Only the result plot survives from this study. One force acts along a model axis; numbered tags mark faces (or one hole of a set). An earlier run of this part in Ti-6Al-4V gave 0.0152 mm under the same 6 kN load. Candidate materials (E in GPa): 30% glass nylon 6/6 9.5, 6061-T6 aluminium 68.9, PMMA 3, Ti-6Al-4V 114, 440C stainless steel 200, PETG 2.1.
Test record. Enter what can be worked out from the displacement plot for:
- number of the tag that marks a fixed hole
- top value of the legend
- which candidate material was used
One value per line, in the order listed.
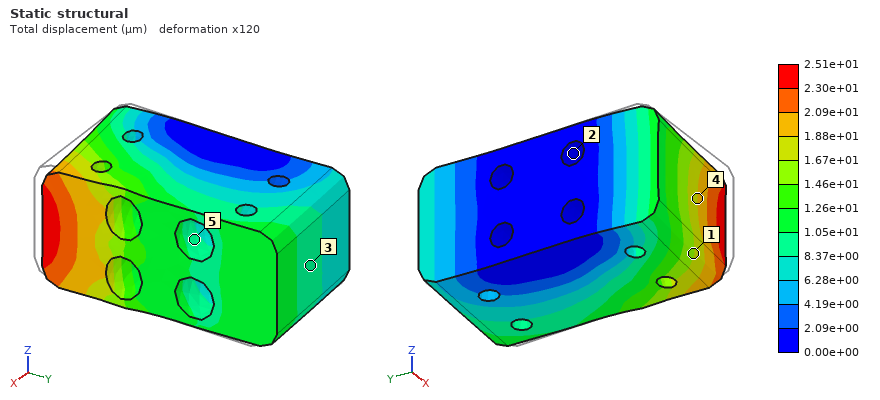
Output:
2
2.51e+01 µm
6061-T6 aluminium
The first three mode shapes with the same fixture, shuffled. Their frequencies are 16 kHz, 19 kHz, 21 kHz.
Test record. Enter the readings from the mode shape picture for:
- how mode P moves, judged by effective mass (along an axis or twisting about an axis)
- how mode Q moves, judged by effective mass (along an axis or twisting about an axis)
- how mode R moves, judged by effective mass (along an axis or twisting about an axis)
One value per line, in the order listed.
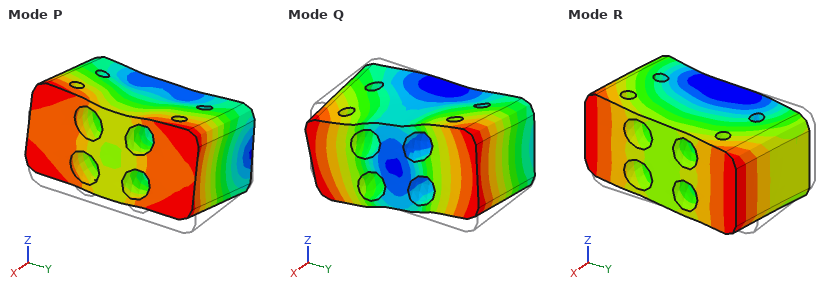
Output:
along Z
twisting about X
along Y
